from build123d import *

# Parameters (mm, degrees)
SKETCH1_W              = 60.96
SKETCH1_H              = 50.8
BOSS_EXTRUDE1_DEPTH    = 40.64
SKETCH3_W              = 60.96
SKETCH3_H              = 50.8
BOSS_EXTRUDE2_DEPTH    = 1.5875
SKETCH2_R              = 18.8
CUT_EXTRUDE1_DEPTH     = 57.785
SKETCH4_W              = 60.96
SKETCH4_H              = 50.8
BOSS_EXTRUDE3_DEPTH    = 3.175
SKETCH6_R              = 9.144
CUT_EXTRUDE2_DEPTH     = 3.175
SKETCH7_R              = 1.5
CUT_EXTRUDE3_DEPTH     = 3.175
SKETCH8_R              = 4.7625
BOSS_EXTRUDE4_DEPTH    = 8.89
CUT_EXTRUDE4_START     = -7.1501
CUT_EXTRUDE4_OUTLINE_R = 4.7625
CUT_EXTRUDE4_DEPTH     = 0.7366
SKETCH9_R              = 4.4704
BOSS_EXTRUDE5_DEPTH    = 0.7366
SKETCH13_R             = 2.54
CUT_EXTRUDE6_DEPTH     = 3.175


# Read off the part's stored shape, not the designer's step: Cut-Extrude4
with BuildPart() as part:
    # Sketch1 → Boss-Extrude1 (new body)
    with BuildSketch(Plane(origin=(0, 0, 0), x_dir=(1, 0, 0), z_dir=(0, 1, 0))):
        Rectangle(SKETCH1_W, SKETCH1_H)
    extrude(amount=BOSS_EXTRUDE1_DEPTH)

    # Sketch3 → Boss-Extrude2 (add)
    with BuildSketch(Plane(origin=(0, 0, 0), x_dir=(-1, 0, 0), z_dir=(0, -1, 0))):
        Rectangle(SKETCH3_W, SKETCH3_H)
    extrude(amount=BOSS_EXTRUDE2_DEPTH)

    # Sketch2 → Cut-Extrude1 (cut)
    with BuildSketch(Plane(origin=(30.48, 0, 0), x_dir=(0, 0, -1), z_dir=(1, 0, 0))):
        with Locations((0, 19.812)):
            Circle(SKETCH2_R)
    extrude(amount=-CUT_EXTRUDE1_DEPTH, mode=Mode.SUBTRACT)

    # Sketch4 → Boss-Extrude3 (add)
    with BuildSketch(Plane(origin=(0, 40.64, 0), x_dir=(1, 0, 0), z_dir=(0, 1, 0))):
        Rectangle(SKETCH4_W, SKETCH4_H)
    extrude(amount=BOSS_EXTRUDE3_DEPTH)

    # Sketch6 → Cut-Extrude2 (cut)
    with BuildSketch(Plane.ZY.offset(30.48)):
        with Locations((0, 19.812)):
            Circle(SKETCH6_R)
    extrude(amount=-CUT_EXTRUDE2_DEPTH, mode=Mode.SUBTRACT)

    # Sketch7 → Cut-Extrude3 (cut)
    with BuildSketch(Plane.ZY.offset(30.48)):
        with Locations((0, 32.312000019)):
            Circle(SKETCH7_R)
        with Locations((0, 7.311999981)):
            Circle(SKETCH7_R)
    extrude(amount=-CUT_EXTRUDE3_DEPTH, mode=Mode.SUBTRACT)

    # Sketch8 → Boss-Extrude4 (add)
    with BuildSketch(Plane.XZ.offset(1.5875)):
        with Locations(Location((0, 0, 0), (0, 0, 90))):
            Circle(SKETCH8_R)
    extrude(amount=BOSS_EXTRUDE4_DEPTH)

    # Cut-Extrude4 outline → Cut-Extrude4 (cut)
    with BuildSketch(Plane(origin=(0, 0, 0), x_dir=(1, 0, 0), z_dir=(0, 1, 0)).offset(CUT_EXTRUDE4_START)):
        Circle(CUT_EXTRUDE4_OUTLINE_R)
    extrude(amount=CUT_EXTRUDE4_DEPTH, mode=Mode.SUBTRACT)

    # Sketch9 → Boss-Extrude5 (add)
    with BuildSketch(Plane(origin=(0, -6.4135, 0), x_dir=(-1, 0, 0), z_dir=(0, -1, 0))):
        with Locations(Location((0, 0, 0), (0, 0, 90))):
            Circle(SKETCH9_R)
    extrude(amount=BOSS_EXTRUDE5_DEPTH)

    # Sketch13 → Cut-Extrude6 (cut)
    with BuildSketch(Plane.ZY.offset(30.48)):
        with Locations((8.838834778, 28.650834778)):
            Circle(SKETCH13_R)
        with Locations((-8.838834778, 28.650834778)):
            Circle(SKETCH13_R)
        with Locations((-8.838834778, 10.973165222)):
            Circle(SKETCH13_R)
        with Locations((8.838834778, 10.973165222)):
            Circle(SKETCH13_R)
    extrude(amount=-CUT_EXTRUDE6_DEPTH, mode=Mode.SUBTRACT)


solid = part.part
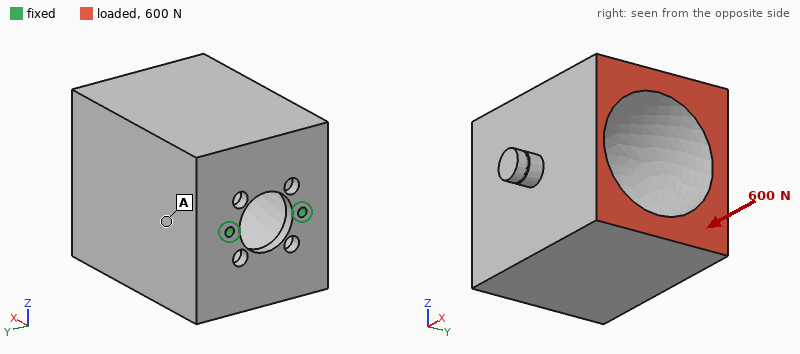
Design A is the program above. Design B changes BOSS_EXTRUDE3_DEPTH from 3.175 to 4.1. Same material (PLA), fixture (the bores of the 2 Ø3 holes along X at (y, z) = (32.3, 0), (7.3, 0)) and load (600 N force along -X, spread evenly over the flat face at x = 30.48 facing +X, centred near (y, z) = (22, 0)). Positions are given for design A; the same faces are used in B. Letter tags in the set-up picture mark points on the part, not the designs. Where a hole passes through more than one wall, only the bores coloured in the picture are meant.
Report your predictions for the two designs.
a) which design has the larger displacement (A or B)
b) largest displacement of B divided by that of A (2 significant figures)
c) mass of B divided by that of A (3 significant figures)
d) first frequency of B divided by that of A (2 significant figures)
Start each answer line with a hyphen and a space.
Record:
- B
- 1.1
- 1.04
- 0.98
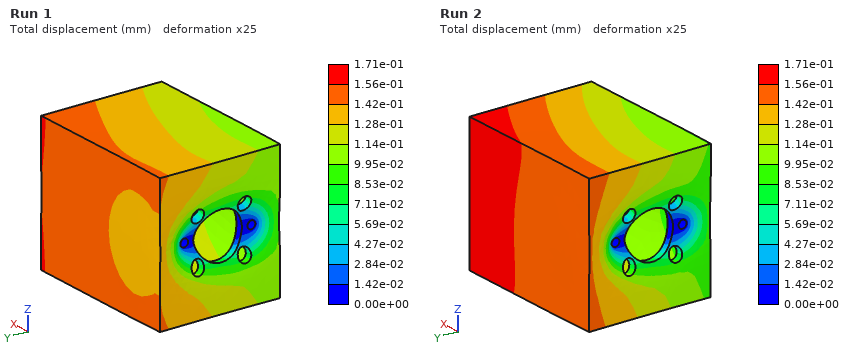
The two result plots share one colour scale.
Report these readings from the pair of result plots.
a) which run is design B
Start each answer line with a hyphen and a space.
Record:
- Run 2
